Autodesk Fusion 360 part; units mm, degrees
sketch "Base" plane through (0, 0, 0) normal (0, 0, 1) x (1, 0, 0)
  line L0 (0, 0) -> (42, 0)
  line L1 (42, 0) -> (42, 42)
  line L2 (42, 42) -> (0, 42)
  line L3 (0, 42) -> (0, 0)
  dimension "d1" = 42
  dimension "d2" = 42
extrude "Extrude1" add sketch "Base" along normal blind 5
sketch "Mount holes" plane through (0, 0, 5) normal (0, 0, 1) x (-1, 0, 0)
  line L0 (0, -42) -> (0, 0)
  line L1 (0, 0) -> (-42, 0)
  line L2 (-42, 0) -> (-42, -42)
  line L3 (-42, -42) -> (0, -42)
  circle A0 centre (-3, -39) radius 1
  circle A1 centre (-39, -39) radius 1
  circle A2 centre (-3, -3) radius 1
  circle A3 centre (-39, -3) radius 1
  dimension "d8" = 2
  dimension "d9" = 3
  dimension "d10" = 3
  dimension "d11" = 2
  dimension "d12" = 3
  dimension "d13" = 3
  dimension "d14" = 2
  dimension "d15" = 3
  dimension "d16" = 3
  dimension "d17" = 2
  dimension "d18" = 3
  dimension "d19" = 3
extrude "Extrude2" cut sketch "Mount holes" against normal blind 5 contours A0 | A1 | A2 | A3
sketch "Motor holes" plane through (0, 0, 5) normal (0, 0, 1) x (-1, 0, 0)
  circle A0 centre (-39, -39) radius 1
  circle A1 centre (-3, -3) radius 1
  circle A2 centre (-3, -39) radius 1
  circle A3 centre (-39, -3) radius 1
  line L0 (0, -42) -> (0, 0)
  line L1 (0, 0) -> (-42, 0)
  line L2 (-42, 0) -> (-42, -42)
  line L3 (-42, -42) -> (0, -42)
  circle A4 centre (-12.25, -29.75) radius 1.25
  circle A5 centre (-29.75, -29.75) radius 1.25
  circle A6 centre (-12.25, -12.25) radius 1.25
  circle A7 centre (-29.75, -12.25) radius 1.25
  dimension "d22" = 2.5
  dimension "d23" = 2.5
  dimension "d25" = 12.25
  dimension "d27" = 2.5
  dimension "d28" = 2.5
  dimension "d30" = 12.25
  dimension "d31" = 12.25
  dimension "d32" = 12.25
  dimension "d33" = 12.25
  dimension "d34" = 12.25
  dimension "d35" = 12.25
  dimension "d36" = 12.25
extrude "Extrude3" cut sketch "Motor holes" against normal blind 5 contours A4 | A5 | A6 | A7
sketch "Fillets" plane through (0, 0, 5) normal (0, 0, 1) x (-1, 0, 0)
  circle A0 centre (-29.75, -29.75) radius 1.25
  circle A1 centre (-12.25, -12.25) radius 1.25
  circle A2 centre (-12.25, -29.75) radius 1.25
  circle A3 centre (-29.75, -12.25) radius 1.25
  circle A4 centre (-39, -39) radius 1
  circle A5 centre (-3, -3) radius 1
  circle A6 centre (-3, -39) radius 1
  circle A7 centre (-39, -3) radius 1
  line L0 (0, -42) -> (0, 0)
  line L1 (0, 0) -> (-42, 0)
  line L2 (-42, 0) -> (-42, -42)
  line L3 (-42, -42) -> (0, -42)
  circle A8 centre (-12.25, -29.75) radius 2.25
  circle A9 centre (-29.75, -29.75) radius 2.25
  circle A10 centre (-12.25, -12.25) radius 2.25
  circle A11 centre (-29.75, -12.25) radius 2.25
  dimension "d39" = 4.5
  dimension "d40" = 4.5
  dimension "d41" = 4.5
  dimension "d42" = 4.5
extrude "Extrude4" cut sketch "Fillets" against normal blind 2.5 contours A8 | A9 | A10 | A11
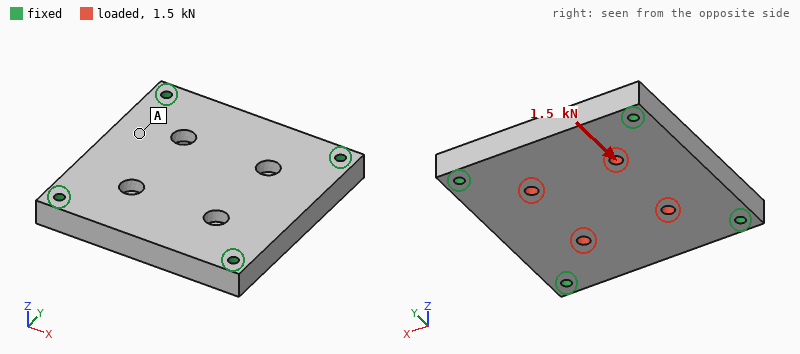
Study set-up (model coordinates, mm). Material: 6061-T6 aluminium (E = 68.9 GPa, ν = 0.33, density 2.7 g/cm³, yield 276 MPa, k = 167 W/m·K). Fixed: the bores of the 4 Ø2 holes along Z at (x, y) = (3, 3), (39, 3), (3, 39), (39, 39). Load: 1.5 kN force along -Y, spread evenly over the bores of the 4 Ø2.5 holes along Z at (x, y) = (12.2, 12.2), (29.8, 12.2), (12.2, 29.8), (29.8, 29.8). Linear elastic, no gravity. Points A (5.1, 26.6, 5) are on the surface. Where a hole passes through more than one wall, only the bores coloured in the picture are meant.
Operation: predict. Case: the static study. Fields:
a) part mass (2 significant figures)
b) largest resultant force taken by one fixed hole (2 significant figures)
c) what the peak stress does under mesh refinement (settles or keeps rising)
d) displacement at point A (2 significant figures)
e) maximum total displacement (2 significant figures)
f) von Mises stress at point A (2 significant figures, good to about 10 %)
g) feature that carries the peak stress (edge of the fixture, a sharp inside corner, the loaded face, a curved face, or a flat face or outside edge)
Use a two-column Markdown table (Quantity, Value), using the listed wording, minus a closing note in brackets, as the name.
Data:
| Quantity | Value |
|---|---|
| part mass | 23 g |
| largest resultant force taken by one fixed hole | 410 N |
| what the peak stress does under mesh refinement | keeps rising |
| displacement at point A | 1.3 µm |
| maximum total displacement | 3.2 µm |
| von Mises stress at point A | 4.3 MPa |
| feature that carries the peak stress | edge of the fixture |
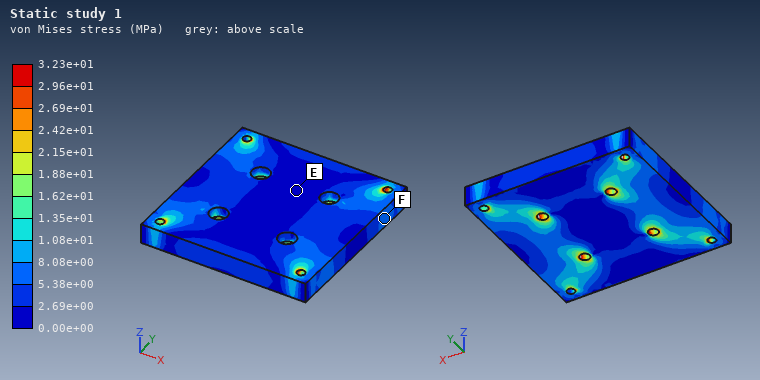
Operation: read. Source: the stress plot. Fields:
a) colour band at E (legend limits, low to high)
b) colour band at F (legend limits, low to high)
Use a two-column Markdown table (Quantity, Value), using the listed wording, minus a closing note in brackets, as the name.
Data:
| Quantity | Value |
|---|---|
| colour band at E | 0.00e+00 to 2.69e+00 MPa |
| colour band at F | 5.38e+00 to 8.08e+00 MPa |
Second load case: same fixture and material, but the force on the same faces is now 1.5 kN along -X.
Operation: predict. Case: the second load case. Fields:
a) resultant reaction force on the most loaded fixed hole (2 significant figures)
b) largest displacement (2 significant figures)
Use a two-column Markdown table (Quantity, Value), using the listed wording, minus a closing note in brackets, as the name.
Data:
| Quantity | Value |
|---|---|
| resultant reaction force on the most loaded fixed hole | 410 N |
| largest displacement | 3.2 µm |
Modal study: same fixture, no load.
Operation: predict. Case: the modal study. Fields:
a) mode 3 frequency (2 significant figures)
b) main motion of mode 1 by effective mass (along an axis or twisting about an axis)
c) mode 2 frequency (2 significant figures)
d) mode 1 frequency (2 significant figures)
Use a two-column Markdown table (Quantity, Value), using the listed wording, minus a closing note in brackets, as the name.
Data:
| Quantity | Value |
|---|---|
| mode 3 frequency | 18 kHz |
| main motion of mode 1 by effective mass | along Z |
| mode 2 frequency | 18 kHz |
| mode 1 frequency | 11 kHz |
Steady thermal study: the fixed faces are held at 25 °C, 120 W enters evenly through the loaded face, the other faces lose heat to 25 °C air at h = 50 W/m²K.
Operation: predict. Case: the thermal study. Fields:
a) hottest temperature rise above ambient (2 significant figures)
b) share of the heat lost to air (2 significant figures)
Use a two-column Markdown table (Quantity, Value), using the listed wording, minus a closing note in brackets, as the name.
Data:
| Quantity | Value |
|---|---|
| hottest temperature rise above ambient | 47 K |
| share of the heat lost to air | 4.5 % |
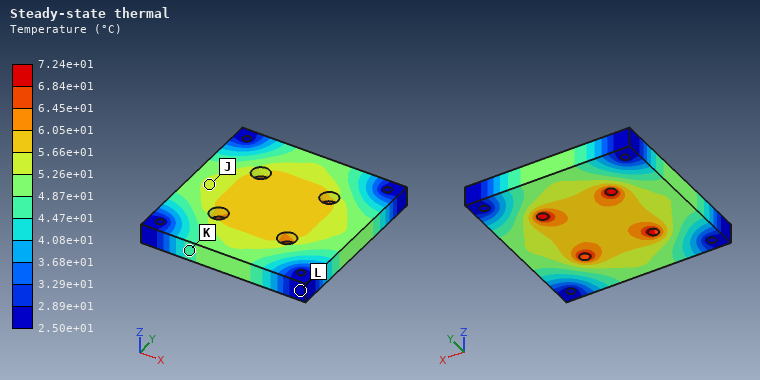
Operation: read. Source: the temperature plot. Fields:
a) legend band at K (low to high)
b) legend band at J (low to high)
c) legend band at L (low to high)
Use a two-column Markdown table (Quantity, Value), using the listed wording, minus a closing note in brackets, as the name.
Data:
| Quantity | Value |
|---|---|
| legend band at K | 4.47e+01 to 4.87e+01 °C |
| legend band at J | 5.26e+01 to 5.66e+01 °C |
| legend band at L | 2.50e+01 to 2.89e+01 °C |
